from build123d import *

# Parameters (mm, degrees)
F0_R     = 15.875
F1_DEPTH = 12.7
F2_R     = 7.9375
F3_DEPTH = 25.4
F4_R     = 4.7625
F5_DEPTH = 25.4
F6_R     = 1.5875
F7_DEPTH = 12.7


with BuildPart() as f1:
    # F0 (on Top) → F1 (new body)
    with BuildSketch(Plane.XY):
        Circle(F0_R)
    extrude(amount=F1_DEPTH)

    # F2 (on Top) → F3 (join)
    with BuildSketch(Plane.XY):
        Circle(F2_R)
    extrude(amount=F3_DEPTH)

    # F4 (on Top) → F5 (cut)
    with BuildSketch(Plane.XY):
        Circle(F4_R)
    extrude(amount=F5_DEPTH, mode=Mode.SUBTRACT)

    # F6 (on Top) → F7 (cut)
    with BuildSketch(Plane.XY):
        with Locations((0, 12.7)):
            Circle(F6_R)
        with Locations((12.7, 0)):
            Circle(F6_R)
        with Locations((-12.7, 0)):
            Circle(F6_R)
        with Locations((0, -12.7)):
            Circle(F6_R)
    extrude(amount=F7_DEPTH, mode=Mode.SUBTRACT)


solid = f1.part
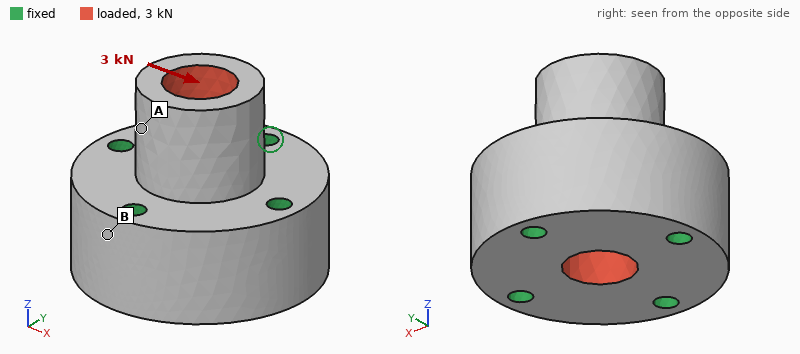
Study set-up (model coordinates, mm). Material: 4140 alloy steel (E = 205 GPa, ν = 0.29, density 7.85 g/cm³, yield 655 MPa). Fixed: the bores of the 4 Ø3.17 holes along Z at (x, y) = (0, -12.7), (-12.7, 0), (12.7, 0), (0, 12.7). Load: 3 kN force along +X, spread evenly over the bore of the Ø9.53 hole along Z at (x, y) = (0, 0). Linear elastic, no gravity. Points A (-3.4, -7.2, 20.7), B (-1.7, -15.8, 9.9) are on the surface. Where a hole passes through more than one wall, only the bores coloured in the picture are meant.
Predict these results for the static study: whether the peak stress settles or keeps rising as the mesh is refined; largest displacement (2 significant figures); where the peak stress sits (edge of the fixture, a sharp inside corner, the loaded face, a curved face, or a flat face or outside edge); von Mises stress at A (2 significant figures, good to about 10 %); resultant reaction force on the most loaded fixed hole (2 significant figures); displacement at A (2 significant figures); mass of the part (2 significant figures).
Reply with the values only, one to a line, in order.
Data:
keeps rising
4.1 µm
a sharp inside corner
11 MPa
1.1 kN
2.7 µm
81 g
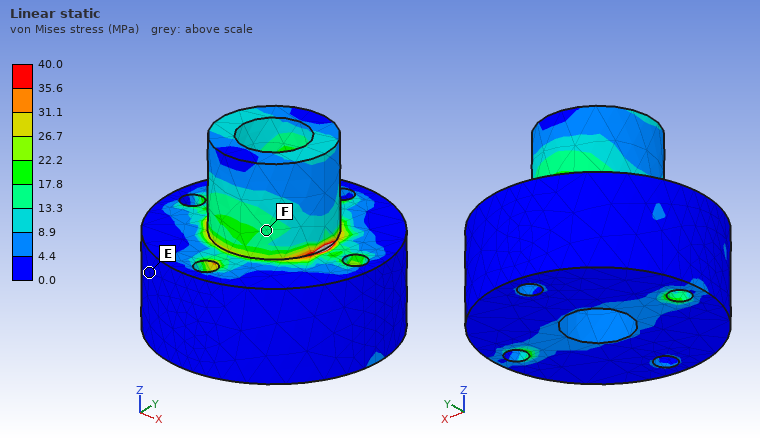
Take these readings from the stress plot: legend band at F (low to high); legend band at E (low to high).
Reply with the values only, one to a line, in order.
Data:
13.3 to 17.8 MPa
0.0 to 4.4 MPa
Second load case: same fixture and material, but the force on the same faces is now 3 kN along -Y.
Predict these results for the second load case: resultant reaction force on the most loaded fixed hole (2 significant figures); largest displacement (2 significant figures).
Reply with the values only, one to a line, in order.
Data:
1.1 kN
4.0 µm
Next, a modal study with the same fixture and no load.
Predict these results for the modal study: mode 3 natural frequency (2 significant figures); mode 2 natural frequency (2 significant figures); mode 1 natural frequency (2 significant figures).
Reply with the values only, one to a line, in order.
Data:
53 kHz
32 kHz
32 kHz
